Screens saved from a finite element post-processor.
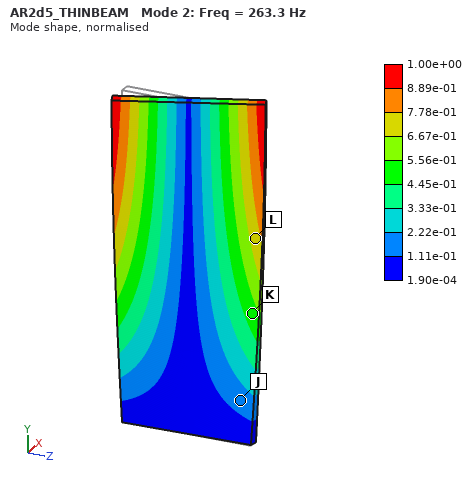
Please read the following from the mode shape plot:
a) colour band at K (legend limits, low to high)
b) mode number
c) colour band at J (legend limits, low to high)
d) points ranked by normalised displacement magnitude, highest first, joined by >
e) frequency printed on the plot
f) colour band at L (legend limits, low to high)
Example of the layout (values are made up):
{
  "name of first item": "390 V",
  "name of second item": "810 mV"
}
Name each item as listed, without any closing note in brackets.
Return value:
{
  "colour band at K": "4.45e-01 to 5.56e-01",
  "mode number": "2",
  "colour band at J": "1.11e-01 to 2.22e-01",
  "points ranked by normalised displacement magnitude, highest first, joined by >": "L > K > J",
  "frequency printed on the plot": "263.3 Hz",
  "colour band at L": "6.67e-01 to 7.78e-01"
}
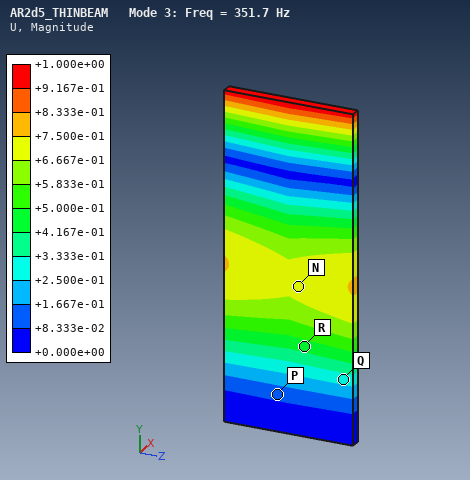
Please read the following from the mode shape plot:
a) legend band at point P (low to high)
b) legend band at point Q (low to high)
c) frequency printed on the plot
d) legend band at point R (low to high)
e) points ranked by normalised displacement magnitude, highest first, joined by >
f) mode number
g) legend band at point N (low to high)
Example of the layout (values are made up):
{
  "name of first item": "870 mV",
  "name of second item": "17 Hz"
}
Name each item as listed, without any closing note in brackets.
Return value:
{
  "legend band at point P": "+8.333e-02 to +1.667e-01",
  "legend band at point Q": "+2.500e-01 to +3.333e-01",
  "frequency printed on the plot": "351.7 Hz",
  "legend band at point R": "+4.167e-01 to +5.000e-01",
  "points ranked by normalised displacement magnitude, highest first, joined by >": "N > R > Q > P",
  "mode number": "3",
  "legend band at point N": "+6.667e-01 to +7.500e-01"
}
